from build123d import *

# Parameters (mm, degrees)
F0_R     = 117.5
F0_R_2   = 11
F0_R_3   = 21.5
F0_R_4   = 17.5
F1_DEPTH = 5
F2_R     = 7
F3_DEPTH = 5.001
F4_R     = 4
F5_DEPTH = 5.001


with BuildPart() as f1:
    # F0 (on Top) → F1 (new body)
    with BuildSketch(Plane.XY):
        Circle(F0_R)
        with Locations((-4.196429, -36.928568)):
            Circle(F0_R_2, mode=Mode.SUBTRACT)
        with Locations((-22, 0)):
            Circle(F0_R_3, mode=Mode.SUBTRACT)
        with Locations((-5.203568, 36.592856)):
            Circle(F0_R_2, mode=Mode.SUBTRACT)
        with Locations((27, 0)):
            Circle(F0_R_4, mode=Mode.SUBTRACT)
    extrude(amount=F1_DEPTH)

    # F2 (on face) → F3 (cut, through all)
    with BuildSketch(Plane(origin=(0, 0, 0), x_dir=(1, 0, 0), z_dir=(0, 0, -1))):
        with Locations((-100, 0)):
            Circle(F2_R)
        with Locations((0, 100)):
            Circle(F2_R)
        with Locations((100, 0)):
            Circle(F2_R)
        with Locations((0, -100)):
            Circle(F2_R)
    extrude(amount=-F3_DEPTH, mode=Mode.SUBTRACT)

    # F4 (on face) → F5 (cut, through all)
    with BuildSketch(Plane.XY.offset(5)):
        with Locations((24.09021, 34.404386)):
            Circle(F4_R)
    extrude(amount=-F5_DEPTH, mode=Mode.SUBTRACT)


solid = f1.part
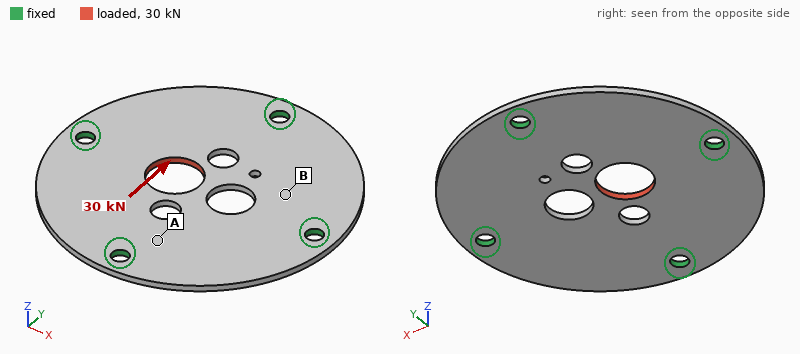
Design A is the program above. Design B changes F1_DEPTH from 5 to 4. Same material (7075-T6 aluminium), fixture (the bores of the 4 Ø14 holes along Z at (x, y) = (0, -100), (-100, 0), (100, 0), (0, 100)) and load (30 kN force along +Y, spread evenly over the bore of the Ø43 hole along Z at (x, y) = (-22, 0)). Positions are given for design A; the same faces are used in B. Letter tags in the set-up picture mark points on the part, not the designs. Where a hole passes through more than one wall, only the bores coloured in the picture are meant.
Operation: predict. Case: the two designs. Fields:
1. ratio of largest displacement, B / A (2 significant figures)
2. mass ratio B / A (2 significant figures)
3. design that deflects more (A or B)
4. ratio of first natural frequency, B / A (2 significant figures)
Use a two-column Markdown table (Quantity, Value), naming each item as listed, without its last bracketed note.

| Quantity | Value |
|---|---|
| ratio of largest displacement, B / A | 1.2 |
| mass ratio B / A | 0.80 |
| design that deflects more | B |
| ratio of first natural frequency, B / A | 0.81 |
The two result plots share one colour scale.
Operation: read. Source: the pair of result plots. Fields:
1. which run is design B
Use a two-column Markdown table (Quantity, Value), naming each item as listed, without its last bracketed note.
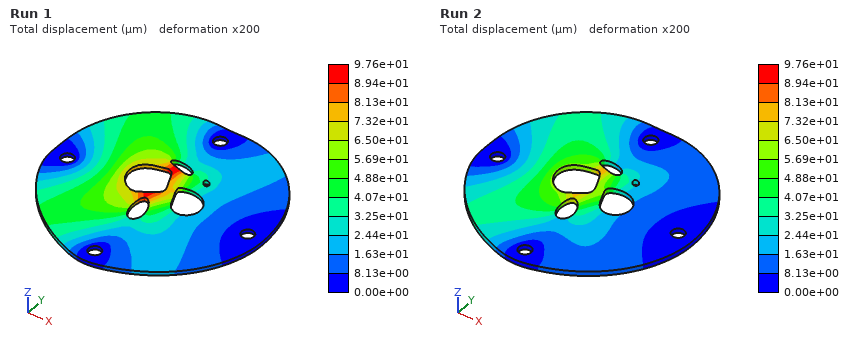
| Quantity | Value |
|---|---|
| which run is design B | Run 1 |
